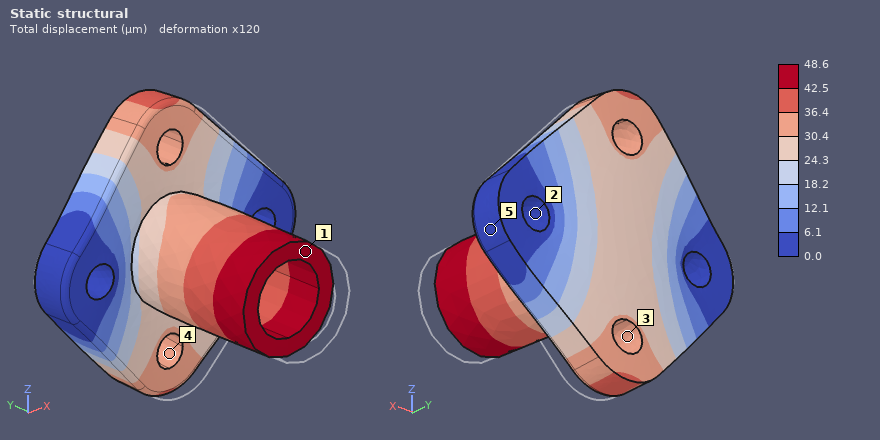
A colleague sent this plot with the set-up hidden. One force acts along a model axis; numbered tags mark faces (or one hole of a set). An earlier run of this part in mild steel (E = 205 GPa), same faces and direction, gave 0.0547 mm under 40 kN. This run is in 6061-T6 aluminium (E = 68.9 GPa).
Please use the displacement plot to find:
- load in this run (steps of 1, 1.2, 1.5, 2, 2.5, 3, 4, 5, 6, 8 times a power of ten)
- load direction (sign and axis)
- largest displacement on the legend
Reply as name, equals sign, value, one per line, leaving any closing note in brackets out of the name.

load in this run = 12 kN
load direction = +Y
largest displacement on the legend = 48.6 µm
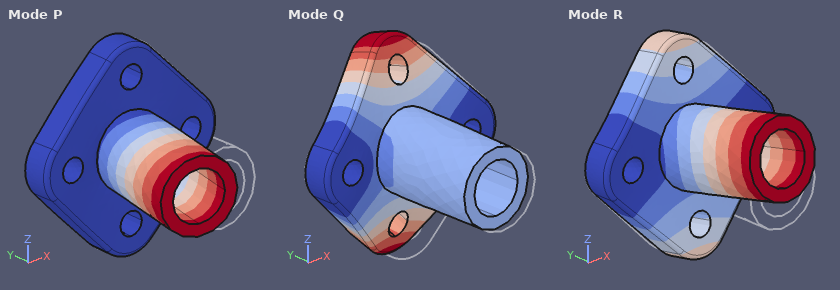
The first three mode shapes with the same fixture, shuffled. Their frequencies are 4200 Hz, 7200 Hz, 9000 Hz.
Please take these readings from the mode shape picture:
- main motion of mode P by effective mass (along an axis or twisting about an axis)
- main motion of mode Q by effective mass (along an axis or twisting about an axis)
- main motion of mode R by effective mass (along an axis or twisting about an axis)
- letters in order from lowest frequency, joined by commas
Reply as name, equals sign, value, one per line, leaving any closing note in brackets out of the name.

main motion of mode P by effective mass = along X
main motion of mode Q by effective mass = along Y
main motion of mode R by effective mass = along Z
letters in order from lowest frequency, joined by commas = R, P, Q
